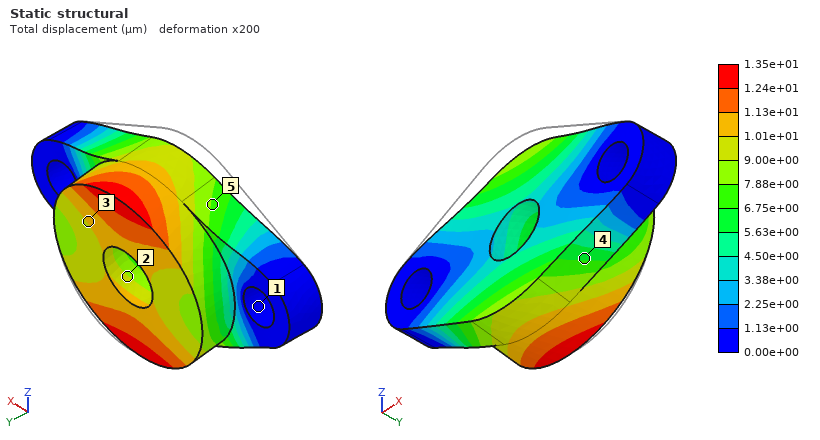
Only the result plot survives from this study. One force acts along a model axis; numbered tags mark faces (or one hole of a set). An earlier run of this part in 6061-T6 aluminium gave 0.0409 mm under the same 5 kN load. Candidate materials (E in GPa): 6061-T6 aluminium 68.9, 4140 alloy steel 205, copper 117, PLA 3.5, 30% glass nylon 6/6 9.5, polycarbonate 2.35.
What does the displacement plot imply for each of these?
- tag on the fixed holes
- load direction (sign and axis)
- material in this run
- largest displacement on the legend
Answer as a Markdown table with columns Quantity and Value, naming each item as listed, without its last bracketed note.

| Quantity | Value |
|---|---|
| tag on the fixed holes | 1 |
| load direction | -Z |
| material in this run | 4140 alloy steel |
| largest displacement on the legend | 1.35e+01 µm |
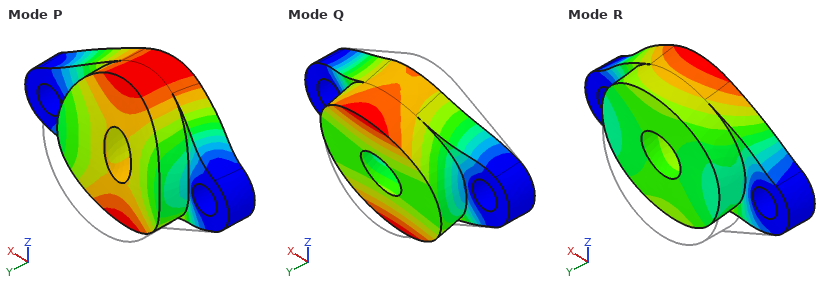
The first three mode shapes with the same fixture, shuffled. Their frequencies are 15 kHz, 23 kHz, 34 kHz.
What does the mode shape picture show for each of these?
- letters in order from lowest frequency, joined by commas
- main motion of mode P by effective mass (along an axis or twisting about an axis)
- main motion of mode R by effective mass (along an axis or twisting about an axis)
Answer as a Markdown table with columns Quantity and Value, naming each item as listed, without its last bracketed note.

| Quantity | Value |
|---|---|
| letters in order from lowest frequency, joined by commas | Q, P, R |
| main motion of mode P by effective mass | along Y |
| main motion of mode R by effective mass | along Z |
